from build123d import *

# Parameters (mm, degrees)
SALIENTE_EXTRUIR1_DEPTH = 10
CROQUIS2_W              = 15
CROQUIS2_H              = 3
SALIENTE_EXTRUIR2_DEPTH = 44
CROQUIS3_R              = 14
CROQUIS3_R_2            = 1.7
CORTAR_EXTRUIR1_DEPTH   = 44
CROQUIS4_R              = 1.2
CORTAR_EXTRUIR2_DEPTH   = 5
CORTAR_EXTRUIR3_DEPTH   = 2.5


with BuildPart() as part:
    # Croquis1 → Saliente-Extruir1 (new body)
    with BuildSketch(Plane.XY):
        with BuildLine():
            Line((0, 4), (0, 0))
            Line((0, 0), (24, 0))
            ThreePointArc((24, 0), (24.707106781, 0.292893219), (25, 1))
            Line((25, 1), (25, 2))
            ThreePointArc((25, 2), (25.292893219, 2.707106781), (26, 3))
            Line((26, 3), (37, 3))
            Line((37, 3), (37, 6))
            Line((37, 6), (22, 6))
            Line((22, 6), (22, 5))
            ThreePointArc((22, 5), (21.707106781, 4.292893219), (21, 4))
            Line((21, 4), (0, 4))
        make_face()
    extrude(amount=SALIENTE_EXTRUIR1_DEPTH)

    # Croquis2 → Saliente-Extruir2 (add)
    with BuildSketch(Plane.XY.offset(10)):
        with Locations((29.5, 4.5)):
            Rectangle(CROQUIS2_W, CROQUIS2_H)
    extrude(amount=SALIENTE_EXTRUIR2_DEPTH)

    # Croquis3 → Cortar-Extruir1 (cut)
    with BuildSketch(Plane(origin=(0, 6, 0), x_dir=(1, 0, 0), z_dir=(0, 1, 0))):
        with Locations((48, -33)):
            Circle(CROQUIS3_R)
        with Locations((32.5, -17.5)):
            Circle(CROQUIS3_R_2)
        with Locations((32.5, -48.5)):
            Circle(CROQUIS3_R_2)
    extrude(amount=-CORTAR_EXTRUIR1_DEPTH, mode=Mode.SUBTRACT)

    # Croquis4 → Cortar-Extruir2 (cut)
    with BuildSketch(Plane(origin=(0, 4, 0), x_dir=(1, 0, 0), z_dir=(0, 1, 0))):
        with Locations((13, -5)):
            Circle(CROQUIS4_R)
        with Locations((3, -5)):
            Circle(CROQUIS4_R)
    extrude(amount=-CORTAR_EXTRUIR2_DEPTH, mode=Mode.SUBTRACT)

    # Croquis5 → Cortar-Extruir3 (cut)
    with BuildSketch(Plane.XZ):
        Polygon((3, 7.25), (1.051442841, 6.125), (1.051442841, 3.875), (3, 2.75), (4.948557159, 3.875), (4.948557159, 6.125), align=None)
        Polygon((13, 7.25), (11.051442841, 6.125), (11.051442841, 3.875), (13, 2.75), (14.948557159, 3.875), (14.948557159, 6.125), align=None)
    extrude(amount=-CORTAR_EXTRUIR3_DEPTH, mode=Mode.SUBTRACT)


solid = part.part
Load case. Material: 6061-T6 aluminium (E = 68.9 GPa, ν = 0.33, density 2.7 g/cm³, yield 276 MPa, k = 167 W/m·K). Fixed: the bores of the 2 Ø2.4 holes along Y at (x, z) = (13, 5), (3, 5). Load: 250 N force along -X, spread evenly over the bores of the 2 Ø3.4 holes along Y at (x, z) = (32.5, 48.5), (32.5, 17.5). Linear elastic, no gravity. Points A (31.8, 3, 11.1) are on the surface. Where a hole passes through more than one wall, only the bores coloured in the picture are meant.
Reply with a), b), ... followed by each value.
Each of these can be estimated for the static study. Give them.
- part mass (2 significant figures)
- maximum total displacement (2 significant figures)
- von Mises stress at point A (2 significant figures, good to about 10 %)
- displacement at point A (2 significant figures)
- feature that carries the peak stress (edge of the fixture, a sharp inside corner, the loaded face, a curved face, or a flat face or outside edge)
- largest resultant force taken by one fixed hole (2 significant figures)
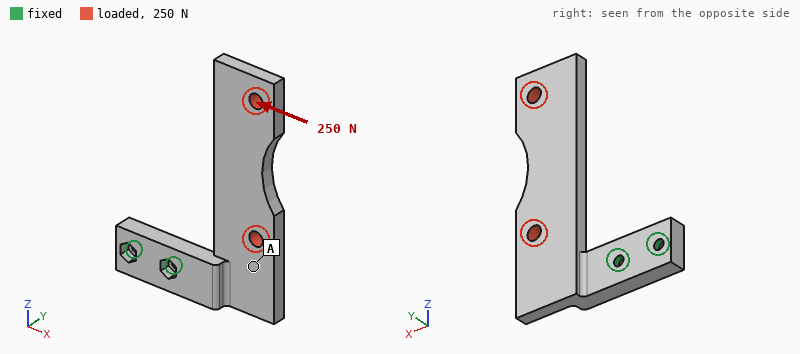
a) 8.5 g
b) 0.52 mm
c) 23 MPa
d) 0.12 mm
e) a curved face
f) 590 N
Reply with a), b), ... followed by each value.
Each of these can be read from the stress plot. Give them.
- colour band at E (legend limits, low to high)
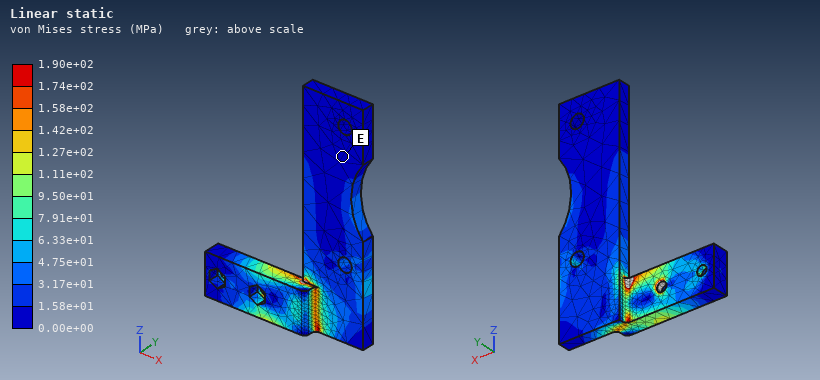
a) 0.00e+00 to 1.58e+01 MPa
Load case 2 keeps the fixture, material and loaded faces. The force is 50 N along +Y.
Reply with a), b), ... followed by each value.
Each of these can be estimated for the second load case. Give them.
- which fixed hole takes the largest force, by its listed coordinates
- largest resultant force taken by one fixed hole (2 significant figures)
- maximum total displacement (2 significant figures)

a) (13, 5)
b) 170 N
c) 0.78 mm
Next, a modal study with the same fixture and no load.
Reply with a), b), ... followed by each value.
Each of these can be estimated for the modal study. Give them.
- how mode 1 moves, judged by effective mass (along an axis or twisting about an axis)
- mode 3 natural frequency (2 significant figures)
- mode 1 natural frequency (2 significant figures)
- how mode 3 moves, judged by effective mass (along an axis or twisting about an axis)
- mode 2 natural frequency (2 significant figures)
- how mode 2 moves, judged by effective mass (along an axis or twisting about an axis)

a) along Y
b) 3200 Hz
c) 760 Hz
d) along Y
e) 2000 Hz
f) along X
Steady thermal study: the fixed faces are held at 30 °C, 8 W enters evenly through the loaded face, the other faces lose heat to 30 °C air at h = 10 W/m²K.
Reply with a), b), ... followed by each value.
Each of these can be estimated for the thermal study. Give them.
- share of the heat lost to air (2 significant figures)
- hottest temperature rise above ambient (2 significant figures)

a) 8.3 %
b) 49 K
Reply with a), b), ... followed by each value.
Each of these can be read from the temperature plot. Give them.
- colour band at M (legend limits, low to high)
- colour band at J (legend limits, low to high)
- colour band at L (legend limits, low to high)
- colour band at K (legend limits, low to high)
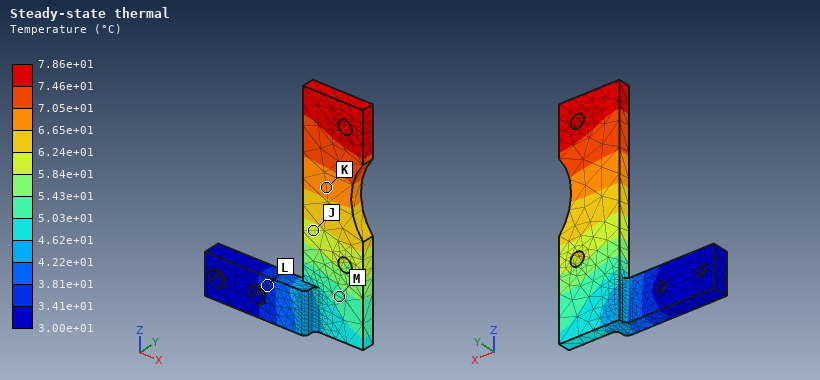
a) 5.03e+01 to 5.43e+01 °C
b) 5.84e+01 to 6.24e+01 °C
c) 3.41e+01 to 3.81e+01 °C
d) 6.65e+01 to 7.05e+01 °C
